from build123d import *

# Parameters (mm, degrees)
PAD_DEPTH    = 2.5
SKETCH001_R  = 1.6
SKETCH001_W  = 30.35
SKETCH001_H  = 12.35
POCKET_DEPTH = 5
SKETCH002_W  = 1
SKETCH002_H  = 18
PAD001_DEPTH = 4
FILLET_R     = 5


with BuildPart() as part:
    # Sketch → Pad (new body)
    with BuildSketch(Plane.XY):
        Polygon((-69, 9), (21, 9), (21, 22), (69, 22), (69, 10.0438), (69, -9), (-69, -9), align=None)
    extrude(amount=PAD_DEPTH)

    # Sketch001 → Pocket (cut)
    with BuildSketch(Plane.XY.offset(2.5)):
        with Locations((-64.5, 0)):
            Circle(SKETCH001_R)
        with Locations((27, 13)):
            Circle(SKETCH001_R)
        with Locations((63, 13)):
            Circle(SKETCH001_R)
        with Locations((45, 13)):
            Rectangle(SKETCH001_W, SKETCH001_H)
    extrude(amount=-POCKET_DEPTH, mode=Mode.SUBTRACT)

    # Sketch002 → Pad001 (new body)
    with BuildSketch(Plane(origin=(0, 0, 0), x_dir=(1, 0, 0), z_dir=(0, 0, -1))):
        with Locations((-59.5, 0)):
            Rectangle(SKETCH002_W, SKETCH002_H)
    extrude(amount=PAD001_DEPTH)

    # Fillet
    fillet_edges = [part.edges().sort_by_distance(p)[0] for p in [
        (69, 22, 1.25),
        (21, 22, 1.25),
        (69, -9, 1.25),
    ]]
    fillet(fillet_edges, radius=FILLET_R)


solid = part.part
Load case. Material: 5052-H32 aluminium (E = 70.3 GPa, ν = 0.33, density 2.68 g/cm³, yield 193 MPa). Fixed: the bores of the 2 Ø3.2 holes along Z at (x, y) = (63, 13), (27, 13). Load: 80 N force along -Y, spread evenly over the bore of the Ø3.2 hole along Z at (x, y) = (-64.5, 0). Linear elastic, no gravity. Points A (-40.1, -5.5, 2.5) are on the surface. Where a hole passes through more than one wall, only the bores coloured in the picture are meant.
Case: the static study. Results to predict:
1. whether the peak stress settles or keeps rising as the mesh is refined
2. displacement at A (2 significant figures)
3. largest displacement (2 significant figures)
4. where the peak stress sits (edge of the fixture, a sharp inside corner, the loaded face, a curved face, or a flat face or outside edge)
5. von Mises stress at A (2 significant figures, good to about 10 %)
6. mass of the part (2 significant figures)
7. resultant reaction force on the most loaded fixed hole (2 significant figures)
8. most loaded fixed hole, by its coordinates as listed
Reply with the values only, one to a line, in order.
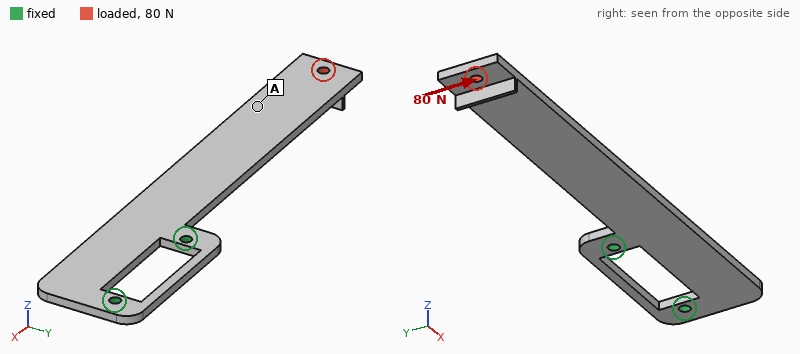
keeps rising
0.20 mm
0.33 mm
a sharp inside corner
9.3 MPa
18 g
310 N
(27, 13)
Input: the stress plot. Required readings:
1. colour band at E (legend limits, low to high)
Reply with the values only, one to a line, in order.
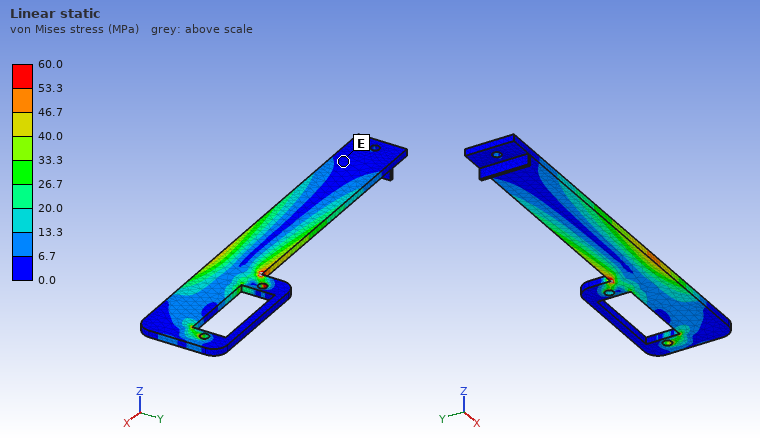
0.0 to 6.7 MPa
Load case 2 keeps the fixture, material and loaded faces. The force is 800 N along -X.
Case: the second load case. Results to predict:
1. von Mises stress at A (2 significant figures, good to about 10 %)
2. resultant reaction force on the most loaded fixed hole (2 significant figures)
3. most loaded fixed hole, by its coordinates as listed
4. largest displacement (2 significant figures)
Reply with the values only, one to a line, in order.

18 MPa
530 N
(27, 13)
94 µm
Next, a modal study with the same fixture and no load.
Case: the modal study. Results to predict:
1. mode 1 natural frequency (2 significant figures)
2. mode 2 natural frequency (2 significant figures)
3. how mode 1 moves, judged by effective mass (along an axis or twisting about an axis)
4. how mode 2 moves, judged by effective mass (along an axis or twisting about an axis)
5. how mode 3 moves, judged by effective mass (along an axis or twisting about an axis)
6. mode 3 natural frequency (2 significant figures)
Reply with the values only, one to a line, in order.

200 Hz
1200 Hz
along Z
along Z
along Y
1400 Hz
